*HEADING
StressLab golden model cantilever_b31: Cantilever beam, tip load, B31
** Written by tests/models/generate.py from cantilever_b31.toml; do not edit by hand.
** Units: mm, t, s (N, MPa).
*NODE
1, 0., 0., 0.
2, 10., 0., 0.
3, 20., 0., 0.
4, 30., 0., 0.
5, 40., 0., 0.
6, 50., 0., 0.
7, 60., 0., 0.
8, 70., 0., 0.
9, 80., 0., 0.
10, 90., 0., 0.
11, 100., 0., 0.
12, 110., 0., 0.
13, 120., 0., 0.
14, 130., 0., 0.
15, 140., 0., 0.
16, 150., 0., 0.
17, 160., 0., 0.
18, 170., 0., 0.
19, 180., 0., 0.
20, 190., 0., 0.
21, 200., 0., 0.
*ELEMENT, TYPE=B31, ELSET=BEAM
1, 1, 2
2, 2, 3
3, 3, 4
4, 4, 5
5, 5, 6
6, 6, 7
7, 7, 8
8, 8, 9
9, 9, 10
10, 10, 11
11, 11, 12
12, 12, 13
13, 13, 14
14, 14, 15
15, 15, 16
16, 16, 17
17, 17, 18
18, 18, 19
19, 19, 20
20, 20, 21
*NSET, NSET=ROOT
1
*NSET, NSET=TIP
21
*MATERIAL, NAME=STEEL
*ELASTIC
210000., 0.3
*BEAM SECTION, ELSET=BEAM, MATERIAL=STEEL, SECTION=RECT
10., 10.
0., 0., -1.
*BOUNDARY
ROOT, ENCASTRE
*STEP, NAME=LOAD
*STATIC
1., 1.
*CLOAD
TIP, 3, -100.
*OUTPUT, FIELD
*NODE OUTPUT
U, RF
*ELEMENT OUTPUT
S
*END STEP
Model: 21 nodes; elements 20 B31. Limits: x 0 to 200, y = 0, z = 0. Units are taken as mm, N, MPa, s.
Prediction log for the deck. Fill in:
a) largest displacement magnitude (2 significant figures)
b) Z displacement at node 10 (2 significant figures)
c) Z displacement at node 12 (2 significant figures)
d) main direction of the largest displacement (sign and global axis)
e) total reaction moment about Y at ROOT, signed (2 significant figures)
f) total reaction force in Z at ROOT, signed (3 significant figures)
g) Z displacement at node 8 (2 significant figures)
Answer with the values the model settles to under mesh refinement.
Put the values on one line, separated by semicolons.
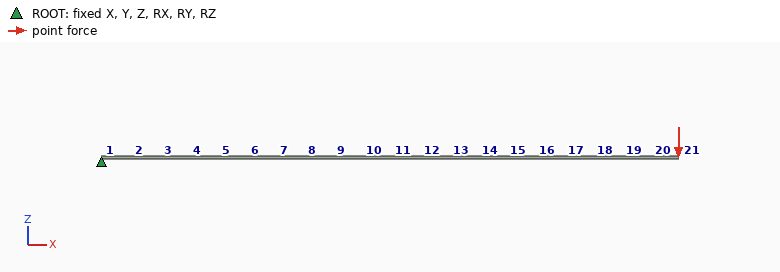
1.5 mm; -0.39 mm; -0.57 mm; -Z; -20000 N·mm; 100 N; -0.25 mm
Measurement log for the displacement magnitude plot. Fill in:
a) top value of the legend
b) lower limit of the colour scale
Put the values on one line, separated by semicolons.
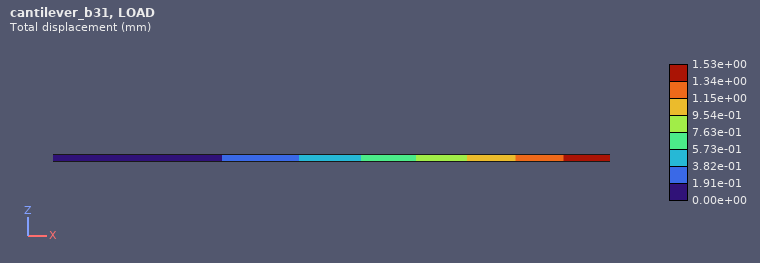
1.53e+00 mm; 0.00e+00 mm
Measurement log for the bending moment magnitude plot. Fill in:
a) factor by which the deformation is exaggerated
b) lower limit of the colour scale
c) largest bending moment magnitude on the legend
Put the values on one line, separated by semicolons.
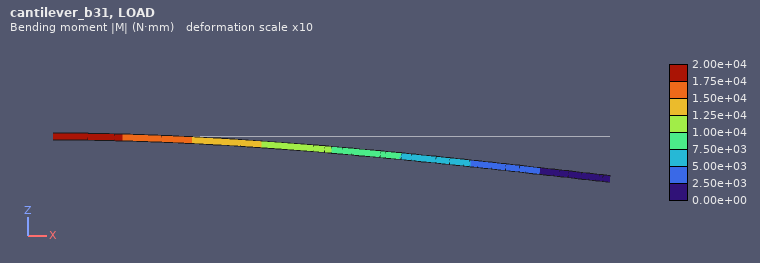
10; 0.00e+00 N·mm; 2.00e+04 N·mm
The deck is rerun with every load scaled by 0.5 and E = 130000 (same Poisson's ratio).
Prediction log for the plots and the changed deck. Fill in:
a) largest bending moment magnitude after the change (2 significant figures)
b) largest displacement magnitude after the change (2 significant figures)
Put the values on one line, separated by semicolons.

10000 N·mm; 1.2 mm
